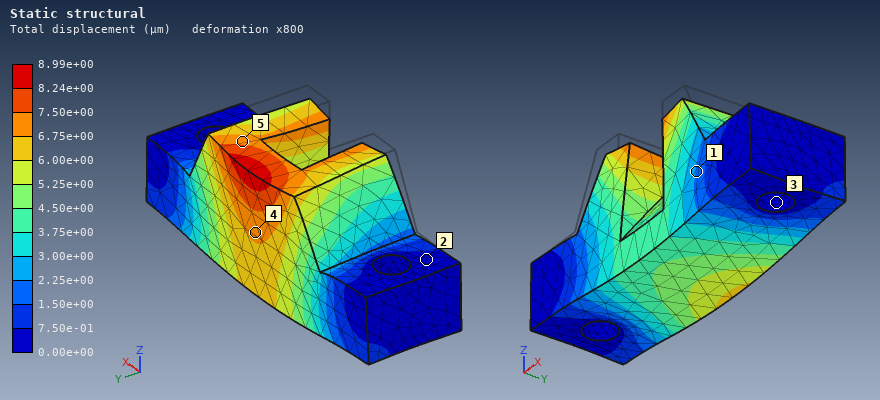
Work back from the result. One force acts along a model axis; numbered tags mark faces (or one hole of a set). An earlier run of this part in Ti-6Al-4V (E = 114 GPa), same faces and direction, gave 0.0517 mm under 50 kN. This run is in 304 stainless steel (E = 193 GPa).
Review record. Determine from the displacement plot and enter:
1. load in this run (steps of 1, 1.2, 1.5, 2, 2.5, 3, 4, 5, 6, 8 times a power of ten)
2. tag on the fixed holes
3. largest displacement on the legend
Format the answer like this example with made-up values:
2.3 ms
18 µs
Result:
15 kN
3
8.99e+00 µm
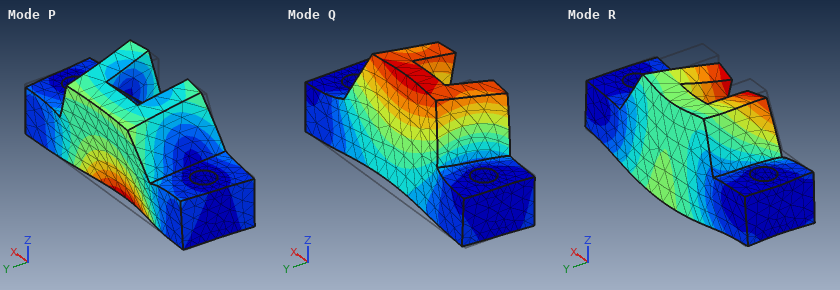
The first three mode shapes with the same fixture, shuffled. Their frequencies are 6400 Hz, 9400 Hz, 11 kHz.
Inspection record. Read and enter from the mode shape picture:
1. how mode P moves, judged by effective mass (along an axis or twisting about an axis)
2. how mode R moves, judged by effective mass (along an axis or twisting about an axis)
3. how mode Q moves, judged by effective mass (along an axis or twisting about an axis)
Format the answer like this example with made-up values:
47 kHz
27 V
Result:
along Y
along Z
along Y
